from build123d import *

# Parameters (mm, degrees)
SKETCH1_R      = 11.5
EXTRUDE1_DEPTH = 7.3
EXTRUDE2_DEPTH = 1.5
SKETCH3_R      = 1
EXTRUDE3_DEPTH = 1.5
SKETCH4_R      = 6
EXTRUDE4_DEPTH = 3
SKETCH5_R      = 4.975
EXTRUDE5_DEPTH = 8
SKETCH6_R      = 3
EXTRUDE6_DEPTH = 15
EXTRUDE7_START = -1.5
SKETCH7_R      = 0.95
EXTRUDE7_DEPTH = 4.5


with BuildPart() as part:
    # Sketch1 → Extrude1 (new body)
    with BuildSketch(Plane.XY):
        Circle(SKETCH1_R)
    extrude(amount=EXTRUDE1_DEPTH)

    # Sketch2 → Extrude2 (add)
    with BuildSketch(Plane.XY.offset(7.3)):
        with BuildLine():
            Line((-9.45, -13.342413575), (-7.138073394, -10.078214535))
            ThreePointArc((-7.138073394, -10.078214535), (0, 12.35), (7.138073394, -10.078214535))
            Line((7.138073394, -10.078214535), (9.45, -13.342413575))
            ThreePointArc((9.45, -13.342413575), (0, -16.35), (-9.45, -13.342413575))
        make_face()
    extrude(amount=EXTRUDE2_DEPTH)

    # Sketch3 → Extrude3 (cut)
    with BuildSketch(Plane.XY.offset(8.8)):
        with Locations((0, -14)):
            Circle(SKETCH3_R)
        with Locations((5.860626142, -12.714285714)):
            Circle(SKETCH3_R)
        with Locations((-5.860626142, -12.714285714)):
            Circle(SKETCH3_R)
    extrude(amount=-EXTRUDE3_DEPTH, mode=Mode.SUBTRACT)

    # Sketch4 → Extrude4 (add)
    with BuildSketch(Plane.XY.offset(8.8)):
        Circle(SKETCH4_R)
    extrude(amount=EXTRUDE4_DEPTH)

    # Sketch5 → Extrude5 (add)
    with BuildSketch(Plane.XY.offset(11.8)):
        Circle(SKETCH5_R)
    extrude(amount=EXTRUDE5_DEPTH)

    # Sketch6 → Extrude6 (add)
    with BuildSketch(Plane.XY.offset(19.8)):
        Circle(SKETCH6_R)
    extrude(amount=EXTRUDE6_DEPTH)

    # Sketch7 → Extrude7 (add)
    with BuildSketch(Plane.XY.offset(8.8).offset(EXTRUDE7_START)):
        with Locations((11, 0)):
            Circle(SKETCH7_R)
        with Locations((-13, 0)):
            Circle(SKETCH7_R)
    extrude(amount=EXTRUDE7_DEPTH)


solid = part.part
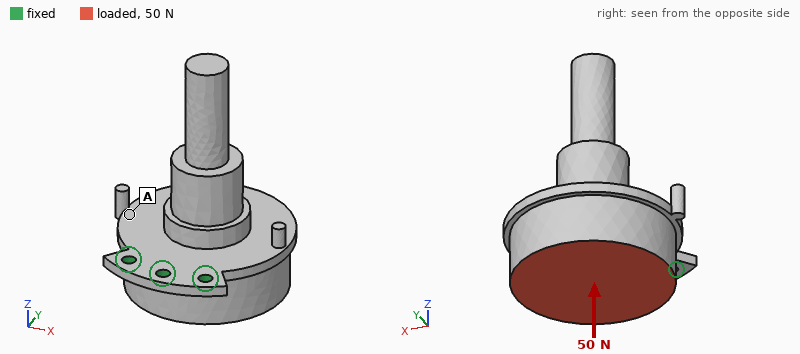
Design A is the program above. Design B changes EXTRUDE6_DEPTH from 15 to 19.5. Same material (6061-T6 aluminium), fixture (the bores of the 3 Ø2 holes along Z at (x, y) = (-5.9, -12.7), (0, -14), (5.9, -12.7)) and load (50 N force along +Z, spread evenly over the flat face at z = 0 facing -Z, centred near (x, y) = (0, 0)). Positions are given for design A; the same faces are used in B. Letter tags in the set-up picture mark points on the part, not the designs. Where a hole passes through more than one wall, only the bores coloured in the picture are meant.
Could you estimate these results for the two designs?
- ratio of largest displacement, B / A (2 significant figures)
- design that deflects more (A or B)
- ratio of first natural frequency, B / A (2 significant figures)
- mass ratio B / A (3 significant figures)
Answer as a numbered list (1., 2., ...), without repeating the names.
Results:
1. 1.1
2. B
3. 0.94
4. 1.02
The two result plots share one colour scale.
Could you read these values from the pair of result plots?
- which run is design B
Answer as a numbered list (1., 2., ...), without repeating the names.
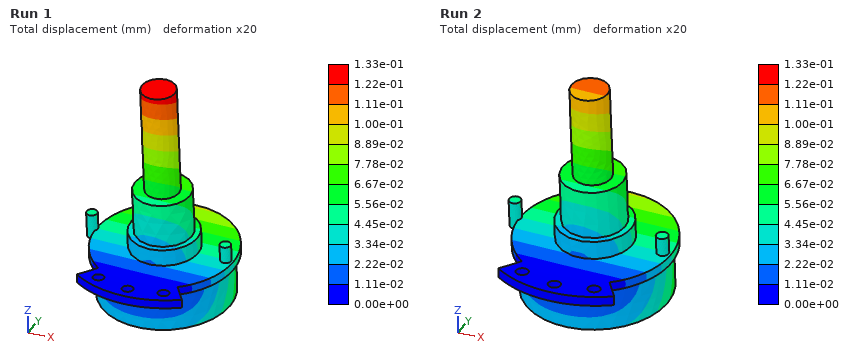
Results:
1. Run 1
